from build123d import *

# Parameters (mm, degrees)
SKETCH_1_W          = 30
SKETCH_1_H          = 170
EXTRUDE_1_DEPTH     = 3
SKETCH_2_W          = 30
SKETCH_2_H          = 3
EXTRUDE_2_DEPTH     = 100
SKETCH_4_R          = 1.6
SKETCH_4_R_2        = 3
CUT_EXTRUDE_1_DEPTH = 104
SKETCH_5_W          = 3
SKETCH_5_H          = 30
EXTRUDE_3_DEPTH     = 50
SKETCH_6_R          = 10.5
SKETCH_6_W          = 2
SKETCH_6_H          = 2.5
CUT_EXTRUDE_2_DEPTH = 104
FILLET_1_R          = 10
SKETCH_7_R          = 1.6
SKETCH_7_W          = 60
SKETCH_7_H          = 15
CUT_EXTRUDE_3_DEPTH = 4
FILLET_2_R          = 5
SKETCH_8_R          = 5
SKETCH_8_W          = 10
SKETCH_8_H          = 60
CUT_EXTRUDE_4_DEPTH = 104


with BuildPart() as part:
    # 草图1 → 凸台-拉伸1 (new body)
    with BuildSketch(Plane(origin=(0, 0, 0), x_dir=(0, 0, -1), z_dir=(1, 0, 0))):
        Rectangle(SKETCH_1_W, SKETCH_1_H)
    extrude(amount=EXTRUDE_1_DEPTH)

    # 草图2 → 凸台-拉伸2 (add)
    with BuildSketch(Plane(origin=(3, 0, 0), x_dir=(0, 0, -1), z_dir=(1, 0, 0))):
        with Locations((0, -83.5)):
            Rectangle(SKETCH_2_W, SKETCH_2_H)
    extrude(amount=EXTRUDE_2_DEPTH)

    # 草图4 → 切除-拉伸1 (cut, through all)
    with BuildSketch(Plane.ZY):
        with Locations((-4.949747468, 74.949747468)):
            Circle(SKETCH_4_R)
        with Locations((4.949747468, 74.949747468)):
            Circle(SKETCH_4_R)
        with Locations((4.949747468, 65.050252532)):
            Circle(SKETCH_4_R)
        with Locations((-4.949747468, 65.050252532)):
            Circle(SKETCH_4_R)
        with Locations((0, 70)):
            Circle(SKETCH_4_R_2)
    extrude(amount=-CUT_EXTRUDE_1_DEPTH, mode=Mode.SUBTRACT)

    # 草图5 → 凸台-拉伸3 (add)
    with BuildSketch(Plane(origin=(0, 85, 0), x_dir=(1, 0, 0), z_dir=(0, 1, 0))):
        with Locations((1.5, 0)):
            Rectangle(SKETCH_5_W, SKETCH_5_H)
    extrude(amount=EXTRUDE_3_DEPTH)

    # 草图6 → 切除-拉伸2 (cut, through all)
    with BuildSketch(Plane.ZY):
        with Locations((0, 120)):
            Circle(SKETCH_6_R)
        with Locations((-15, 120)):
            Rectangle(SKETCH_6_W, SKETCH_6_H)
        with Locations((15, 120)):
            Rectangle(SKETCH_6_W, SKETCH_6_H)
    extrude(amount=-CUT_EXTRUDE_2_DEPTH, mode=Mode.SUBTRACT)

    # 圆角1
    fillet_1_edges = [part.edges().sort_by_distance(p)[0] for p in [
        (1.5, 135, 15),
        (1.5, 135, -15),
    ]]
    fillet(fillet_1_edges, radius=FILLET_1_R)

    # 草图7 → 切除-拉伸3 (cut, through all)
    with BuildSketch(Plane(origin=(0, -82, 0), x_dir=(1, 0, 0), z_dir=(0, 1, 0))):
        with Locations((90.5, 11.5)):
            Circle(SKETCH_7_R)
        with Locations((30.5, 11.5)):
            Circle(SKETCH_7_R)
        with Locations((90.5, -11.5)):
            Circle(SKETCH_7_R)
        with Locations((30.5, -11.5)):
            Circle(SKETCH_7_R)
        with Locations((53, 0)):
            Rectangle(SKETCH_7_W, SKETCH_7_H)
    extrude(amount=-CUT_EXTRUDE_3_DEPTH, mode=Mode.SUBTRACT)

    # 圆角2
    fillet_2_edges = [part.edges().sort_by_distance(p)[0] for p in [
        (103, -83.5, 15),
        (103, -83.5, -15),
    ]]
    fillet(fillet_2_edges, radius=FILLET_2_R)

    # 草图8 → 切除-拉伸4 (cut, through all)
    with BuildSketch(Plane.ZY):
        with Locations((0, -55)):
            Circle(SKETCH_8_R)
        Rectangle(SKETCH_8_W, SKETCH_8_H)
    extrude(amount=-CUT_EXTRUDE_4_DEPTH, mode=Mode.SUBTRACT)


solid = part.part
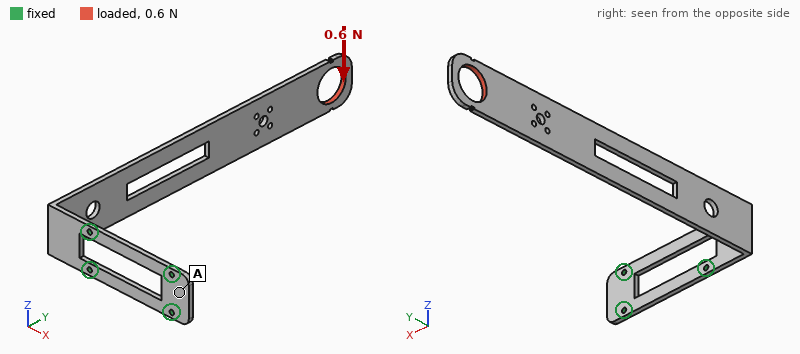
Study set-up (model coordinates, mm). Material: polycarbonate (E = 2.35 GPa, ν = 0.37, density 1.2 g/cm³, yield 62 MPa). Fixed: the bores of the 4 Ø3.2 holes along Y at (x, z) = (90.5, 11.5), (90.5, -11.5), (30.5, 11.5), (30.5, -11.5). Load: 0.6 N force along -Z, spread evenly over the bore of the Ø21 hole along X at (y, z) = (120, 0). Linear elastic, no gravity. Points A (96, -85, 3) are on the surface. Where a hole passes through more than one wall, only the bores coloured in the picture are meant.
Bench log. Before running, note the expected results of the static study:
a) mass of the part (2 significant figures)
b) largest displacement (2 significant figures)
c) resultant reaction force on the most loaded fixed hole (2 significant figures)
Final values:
27 g
2.3 mm
4.5 N
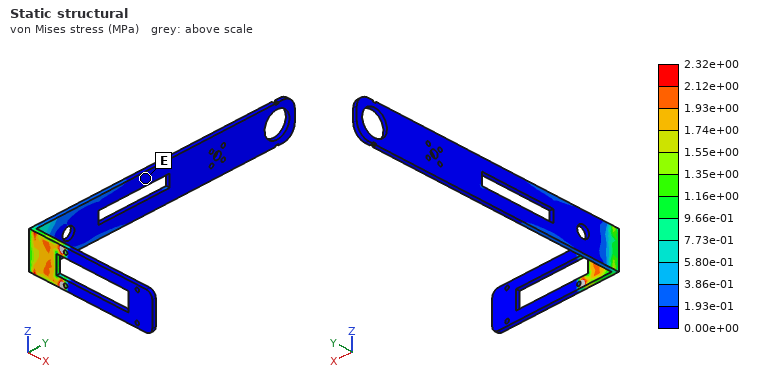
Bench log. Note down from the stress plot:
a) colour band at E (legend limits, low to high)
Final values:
0.00e+00 to 1.93e-01 MPa
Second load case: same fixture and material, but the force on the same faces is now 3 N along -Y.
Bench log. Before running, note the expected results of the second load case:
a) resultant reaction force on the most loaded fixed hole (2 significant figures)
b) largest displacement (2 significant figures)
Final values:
1.5 N
2.5 mm
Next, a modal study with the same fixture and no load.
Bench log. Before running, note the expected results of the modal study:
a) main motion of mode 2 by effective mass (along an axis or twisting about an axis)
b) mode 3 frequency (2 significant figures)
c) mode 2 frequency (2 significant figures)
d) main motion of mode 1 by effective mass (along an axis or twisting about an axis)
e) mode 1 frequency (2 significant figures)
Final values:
along Z
77 Hz
31 Hz
along X
12 Hz
